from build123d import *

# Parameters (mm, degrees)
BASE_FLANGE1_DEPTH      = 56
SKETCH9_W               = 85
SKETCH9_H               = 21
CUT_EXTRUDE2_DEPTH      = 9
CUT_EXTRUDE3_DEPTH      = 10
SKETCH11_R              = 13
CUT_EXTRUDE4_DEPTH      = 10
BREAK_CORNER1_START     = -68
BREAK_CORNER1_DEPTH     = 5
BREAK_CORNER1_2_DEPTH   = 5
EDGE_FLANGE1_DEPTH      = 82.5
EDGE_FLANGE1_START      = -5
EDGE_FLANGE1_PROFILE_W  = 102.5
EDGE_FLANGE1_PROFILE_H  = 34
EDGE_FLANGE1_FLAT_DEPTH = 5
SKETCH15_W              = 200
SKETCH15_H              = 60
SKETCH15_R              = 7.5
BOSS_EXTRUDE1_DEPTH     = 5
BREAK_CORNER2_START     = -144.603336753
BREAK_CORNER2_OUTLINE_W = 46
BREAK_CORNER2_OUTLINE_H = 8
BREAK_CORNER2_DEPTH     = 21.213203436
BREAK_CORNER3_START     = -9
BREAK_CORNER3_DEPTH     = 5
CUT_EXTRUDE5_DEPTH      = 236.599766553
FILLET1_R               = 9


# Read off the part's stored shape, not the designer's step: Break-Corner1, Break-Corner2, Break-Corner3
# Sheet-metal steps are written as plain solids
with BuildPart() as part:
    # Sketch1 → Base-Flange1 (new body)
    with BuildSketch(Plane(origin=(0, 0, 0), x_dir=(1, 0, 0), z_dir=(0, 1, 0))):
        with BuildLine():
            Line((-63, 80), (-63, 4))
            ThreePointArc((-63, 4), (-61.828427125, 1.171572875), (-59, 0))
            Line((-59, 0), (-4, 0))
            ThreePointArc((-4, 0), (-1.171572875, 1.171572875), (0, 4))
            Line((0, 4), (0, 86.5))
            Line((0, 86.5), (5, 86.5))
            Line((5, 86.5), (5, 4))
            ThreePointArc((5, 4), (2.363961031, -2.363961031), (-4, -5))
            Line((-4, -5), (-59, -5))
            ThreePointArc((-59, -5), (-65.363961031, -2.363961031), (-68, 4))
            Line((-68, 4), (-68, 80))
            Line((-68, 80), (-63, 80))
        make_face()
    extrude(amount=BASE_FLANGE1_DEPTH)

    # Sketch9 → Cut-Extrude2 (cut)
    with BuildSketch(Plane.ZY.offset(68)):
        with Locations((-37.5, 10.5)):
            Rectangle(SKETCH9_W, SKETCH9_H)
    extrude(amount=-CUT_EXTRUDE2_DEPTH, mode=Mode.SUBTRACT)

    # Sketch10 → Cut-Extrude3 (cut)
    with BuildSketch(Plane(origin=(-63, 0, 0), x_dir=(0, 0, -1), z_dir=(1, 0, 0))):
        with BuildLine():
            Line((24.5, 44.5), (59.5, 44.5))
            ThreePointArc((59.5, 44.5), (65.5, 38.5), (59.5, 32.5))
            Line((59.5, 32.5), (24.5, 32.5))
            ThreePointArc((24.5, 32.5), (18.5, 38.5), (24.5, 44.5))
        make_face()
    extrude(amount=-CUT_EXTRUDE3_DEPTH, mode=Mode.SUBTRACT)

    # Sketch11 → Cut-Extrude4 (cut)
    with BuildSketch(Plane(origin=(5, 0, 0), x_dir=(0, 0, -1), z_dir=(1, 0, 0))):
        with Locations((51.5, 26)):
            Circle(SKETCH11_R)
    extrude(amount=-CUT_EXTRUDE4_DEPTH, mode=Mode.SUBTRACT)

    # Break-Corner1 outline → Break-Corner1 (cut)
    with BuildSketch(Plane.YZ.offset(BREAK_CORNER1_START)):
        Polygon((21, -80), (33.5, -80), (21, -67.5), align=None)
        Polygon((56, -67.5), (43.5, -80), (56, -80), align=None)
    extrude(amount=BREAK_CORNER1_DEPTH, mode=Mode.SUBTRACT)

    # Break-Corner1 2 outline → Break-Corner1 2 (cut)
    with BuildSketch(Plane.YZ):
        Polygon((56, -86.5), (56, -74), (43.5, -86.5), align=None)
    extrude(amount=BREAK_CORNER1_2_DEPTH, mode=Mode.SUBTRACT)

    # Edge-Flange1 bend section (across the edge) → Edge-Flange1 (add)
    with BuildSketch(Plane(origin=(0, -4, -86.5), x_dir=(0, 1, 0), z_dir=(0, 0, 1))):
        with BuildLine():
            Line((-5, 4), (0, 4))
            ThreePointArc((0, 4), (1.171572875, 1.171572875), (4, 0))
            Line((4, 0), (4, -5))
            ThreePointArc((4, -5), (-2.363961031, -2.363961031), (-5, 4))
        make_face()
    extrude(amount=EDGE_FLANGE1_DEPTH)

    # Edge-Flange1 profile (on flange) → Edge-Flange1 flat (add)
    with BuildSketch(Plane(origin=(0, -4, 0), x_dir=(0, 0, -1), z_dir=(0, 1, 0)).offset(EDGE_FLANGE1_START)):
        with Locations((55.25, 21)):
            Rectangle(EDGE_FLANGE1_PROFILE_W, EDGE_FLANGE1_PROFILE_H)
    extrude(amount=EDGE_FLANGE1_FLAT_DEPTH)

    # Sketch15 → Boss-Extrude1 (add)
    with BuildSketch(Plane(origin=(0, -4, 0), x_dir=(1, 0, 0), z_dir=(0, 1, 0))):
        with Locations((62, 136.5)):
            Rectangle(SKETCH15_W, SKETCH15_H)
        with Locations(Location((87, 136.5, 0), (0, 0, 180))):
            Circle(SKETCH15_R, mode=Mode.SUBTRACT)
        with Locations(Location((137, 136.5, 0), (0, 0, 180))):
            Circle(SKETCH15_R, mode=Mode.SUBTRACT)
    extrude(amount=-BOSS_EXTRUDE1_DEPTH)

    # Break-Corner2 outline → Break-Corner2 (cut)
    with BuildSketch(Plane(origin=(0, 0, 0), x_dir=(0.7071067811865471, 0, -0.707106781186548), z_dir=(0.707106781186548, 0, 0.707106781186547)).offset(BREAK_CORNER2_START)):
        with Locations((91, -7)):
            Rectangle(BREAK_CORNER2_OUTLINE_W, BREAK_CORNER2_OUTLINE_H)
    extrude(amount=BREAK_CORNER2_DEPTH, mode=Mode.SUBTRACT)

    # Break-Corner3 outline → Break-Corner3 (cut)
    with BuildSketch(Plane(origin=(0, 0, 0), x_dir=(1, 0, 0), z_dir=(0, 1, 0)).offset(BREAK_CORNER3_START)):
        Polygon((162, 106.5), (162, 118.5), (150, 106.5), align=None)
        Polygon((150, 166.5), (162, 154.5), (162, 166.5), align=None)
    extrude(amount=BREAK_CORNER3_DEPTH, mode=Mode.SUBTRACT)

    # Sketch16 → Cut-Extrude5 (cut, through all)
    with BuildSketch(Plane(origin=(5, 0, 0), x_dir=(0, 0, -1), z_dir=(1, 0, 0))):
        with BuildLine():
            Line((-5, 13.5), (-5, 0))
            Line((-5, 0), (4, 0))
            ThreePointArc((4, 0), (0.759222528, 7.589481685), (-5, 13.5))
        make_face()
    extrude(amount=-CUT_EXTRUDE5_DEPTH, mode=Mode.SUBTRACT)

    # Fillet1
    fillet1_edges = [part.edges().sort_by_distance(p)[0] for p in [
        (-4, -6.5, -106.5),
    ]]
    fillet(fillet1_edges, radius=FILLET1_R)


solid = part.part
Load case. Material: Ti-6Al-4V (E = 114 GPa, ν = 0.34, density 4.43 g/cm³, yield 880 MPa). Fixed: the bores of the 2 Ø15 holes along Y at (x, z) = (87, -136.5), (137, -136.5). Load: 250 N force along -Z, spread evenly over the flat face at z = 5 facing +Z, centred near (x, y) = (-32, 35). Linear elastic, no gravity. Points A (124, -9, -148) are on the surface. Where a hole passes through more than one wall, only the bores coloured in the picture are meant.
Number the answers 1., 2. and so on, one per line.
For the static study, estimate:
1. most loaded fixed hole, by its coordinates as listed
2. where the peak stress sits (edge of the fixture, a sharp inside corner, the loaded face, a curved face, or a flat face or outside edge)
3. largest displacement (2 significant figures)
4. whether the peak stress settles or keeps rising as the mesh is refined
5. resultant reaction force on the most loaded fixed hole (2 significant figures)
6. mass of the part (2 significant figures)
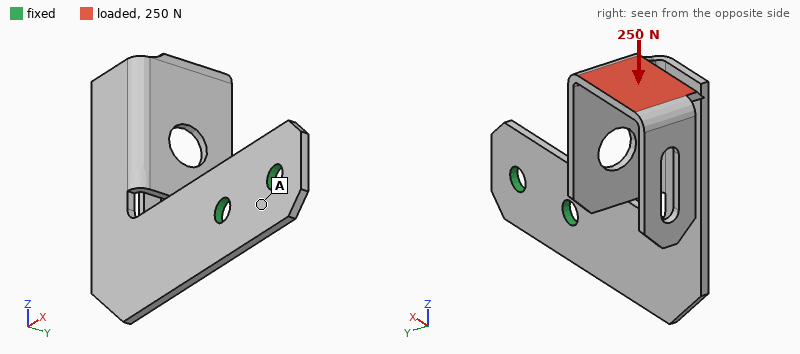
1. (87, -136.5)
2. a sharp inside corner
3. 3.1 mm
4. keeps rising
5. 600 N
6. 550 g
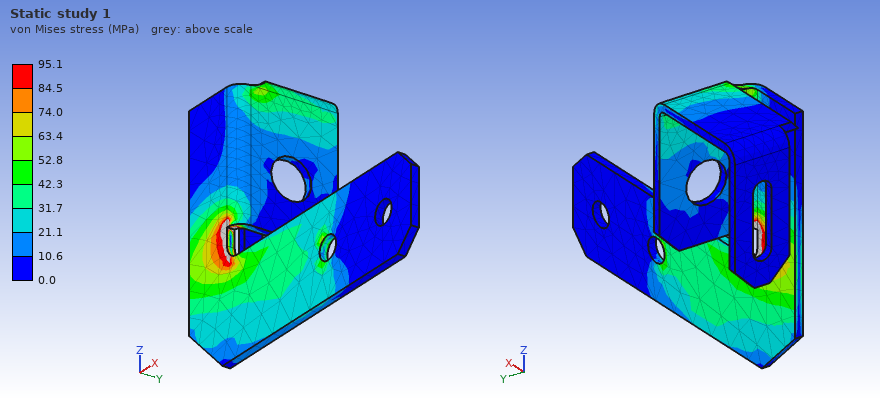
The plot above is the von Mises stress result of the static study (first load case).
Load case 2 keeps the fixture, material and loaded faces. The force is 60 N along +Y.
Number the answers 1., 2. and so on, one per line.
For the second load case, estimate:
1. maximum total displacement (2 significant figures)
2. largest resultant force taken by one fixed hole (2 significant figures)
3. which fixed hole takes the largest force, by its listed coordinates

1. 2.7 mm
2. 73 N
3. (87, -136.5)
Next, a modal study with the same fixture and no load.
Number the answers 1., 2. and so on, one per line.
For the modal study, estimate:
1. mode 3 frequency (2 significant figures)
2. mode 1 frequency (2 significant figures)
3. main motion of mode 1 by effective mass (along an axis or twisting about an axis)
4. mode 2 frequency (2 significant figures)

1. 240 Hz
2. 60 Hz
3. along Y
4. 130 Hz
